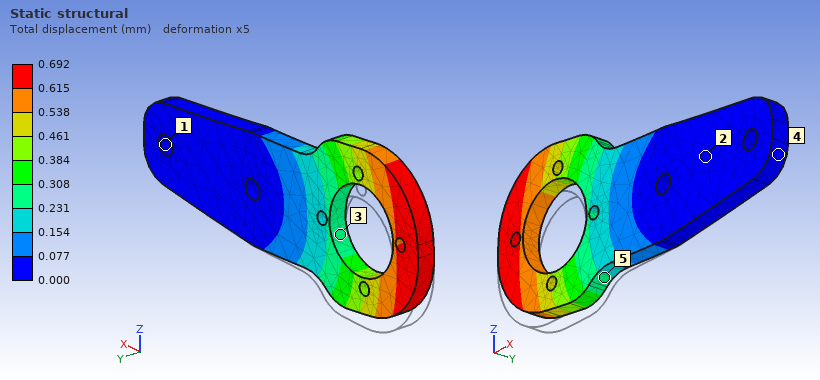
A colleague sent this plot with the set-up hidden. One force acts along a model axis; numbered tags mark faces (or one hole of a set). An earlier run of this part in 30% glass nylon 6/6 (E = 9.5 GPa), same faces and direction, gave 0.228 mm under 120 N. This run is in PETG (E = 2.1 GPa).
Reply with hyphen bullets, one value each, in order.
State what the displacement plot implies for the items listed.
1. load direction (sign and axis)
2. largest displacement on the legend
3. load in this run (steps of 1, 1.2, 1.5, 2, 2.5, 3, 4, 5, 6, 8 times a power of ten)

- +Z
- 0.692 mm
- 80 N
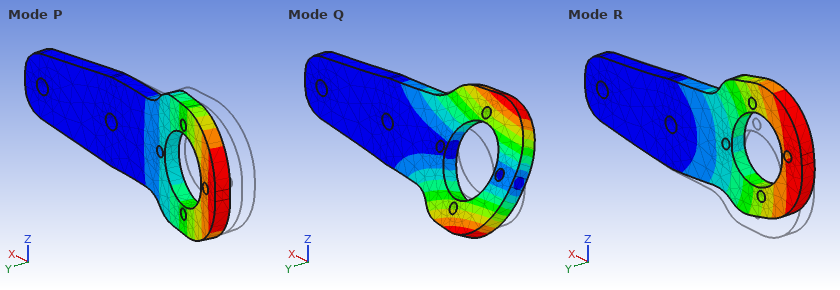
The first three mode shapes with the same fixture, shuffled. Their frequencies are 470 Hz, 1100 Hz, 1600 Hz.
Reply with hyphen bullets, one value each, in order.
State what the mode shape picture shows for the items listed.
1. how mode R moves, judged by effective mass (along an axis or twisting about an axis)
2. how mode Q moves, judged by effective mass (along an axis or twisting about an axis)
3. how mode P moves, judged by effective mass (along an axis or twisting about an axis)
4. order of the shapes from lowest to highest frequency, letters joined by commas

- along Z
- twisting about X
- along Y
- P, Q, R
